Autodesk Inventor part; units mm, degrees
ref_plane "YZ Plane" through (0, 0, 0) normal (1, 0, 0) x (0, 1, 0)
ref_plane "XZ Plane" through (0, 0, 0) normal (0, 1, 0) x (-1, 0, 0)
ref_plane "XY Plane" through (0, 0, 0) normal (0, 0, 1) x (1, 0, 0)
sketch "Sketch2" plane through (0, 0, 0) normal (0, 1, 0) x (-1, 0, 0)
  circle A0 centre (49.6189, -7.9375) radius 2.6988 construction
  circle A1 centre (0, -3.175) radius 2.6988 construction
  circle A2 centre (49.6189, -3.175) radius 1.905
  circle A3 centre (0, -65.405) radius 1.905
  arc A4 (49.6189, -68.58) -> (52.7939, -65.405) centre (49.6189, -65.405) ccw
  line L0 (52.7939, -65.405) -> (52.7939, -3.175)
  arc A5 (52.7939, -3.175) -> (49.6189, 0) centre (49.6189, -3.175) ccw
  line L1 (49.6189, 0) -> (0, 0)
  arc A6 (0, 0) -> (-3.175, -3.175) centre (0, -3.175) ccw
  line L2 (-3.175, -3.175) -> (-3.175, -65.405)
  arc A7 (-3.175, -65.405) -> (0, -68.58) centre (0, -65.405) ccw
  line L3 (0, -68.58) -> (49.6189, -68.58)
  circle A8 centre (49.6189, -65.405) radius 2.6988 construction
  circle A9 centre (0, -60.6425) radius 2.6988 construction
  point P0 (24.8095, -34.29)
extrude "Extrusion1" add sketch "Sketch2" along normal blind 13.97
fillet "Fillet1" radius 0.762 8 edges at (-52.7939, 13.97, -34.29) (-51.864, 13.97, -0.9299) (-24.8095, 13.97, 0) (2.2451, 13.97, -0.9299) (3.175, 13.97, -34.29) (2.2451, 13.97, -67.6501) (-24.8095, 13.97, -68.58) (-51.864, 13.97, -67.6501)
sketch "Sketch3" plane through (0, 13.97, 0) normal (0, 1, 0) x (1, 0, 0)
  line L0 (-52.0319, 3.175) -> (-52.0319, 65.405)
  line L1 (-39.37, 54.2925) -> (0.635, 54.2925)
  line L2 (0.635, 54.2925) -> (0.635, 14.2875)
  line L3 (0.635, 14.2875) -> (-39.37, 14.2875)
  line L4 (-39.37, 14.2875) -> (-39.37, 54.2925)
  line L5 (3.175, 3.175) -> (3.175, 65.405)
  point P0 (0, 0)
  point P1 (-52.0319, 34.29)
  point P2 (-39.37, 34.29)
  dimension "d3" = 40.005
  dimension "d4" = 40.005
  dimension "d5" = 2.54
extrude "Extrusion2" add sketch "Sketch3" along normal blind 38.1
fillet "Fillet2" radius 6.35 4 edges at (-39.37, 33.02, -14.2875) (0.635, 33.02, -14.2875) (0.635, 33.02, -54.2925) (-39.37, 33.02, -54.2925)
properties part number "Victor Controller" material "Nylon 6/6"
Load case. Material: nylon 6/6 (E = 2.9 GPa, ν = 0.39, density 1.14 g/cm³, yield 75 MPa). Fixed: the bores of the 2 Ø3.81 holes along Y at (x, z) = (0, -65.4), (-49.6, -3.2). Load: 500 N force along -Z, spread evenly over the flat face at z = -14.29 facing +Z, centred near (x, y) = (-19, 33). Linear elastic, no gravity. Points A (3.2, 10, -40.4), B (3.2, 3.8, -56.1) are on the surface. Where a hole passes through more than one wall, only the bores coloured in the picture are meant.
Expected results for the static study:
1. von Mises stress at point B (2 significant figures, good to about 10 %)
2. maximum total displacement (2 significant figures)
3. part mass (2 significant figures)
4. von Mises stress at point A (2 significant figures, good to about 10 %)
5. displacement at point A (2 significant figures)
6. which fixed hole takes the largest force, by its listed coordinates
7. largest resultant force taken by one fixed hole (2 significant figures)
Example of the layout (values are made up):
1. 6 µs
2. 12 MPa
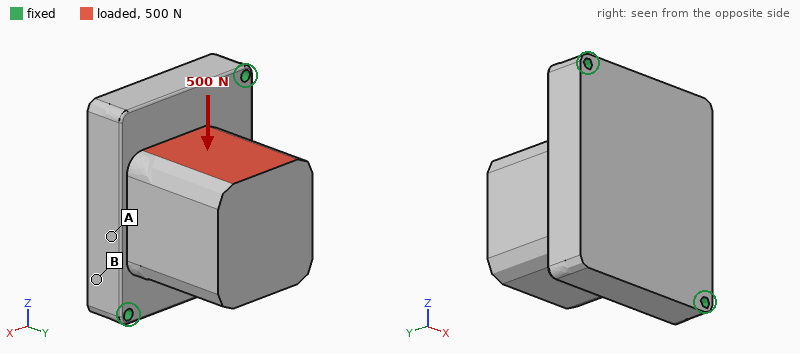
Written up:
1. 4.3 MPa
2. 0.40 mm
3. 130 g
4. 1.8 MPa
5. 0.12 mm
6. (0, -65.4)
7. 320 N
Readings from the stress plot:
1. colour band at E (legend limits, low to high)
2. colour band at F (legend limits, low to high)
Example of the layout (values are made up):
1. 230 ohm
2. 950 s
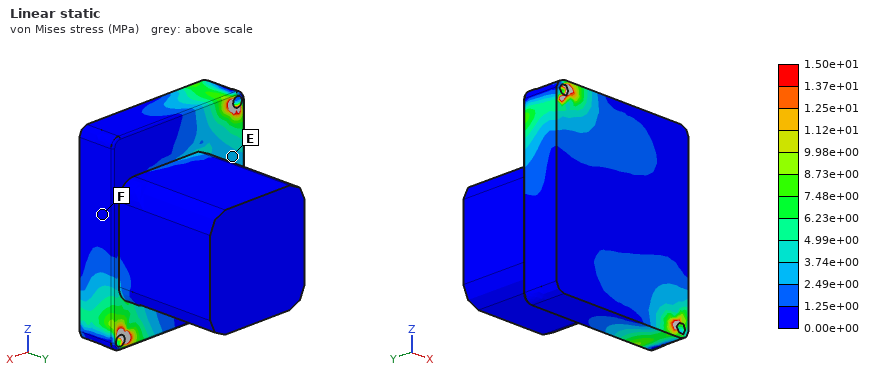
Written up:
1. 2.49e+00 to 3.74e+00 MPa
2. 0.00e+00 to 1.25e+00 MPa
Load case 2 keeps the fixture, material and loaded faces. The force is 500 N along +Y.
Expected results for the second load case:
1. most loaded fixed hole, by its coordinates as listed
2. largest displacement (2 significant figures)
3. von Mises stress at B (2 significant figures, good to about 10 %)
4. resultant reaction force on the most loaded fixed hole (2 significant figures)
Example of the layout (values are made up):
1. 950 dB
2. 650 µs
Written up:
1. (-49.6, -3.2)
2. 0.42 mm
3. 7.6 MPa
4. 350 N
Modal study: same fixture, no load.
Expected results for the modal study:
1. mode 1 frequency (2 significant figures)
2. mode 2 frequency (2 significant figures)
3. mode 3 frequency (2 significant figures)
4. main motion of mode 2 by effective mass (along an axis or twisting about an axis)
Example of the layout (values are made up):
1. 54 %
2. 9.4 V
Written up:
1. 580 Hz
2. 1500 Hz
3. 2000 Hz
4. along Y
